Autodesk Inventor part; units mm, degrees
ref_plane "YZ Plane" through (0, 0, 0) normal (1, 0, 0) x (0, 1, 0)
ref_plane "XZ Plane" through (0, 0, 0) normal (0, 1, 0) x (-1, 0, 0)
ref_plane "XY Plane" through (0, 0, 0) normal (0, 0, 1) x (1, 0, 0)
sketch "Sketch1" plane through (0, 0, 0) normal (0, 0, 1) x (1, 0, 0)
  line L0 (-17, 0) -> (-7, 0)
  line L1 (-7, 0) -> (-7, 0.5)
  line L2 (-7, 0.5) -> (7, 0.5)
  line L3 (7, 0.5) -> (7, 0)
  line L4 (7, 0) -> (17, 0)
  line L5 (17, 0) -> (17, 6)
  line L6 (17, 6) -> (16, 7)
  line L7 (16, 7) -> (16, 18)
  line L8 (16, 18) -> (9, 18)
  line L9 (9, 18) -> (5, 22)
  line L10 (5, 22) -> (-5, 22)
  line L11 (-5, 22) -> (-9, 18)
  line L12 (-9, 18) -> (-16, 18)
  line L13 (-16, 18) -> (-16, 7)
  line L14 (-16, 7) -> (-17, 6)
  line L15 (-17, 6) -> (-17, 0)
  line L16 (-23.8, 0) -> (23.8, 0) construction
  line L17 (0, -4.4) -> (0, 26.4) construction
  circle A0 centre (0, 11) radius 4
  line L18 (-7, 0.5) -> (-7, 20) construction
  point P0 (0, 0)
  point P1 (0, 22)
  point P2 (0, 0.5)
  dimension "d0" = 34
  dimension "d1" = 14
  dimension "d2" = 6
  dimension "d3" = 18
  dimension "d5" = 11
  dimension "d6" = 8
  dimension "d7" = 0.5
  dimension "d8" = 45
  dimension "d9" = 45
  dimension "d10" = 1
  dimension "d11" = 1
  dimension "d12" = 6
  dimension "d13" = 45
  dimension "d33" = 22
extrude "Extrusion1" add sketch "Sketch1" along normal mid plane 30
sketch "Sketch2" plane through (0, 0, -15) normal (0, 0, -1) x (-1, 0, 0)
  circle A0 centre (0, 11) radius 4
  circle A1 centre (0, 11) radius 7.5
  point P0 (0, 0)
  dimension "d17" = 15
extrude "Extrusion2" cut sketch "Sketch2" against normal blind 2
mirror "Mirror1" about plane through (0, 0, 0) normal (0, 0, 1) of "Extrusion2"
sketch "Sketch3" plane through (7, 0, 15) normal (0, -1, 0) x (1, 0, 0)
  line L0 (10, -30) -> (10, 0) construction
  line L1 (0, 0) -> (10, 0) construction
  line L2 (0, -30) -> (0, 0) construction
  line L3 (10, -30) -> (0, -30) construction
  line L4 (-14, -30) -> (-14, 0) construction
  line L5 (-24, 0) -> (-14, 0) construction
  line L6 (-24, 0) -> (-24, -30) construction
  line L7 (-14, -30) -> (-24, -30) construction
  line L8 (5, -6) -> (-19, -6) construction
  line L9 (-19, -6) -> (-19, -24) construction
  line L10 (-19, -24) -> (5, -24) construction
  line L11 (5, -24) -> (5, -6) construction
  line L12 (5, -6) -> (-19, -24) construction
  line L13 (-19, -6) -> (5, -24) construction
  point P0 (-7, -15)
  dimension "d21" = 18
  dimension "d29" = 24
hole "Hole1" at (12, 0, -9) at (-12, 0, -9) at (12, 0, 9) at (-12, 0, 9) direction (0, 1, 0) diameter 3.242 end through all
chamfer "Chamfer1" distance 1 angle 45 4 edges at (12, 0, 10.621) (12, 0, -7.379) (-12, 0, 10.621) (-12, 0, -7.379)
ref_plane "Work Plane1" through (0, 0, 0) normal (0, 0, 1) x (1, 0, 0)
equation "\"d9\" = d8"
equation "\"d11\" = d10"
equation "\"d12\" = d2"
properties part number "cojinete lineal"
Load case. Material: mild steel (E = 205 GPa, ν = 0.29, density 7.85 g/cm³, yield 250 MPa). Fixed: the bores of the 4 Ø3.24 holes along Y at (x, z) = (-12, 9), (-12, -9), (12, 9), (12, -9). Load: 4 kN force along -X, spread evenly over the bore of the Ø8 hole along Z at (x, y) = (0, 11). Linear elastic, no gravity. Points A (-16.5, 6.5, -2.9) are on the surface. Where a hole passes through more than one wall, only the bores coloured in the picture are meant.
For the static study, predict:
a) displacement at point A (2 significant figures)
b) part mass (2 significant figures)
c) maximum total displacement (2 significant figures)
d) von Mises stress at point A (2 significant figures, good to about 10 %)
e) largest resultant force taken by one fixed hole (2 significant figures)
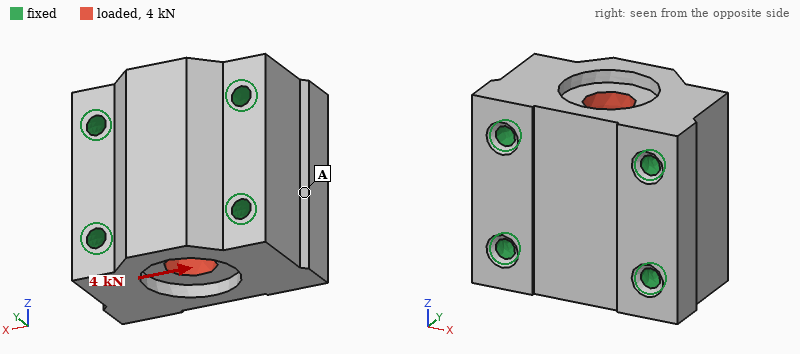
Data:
0.14 µm
130 g
0.42 µm
2.1 MPa
1.0 kN
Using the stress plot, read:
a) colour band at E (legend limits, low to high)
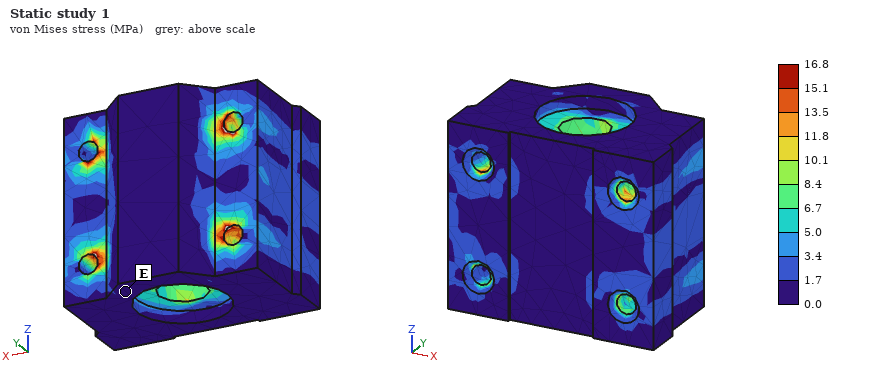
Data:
0.0 to 1.7 MPa
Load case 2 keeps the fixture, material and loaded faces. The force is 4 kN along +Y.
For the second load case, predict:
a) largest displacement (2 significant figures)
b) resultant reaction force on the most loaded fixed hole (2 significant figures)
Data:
0.77 µm
1.0 kN
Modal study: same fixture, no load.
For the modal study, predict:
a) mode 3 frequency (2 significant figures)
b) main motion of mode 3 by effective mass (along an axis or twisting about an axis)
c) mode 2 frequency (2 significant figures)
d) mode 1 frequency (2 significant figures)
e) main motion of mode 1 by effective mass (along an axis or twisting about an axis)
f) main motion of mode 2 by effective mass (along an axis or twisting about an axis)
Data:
63 kHz
along Z
54 kHz
52 kHz
along Z
along Y
